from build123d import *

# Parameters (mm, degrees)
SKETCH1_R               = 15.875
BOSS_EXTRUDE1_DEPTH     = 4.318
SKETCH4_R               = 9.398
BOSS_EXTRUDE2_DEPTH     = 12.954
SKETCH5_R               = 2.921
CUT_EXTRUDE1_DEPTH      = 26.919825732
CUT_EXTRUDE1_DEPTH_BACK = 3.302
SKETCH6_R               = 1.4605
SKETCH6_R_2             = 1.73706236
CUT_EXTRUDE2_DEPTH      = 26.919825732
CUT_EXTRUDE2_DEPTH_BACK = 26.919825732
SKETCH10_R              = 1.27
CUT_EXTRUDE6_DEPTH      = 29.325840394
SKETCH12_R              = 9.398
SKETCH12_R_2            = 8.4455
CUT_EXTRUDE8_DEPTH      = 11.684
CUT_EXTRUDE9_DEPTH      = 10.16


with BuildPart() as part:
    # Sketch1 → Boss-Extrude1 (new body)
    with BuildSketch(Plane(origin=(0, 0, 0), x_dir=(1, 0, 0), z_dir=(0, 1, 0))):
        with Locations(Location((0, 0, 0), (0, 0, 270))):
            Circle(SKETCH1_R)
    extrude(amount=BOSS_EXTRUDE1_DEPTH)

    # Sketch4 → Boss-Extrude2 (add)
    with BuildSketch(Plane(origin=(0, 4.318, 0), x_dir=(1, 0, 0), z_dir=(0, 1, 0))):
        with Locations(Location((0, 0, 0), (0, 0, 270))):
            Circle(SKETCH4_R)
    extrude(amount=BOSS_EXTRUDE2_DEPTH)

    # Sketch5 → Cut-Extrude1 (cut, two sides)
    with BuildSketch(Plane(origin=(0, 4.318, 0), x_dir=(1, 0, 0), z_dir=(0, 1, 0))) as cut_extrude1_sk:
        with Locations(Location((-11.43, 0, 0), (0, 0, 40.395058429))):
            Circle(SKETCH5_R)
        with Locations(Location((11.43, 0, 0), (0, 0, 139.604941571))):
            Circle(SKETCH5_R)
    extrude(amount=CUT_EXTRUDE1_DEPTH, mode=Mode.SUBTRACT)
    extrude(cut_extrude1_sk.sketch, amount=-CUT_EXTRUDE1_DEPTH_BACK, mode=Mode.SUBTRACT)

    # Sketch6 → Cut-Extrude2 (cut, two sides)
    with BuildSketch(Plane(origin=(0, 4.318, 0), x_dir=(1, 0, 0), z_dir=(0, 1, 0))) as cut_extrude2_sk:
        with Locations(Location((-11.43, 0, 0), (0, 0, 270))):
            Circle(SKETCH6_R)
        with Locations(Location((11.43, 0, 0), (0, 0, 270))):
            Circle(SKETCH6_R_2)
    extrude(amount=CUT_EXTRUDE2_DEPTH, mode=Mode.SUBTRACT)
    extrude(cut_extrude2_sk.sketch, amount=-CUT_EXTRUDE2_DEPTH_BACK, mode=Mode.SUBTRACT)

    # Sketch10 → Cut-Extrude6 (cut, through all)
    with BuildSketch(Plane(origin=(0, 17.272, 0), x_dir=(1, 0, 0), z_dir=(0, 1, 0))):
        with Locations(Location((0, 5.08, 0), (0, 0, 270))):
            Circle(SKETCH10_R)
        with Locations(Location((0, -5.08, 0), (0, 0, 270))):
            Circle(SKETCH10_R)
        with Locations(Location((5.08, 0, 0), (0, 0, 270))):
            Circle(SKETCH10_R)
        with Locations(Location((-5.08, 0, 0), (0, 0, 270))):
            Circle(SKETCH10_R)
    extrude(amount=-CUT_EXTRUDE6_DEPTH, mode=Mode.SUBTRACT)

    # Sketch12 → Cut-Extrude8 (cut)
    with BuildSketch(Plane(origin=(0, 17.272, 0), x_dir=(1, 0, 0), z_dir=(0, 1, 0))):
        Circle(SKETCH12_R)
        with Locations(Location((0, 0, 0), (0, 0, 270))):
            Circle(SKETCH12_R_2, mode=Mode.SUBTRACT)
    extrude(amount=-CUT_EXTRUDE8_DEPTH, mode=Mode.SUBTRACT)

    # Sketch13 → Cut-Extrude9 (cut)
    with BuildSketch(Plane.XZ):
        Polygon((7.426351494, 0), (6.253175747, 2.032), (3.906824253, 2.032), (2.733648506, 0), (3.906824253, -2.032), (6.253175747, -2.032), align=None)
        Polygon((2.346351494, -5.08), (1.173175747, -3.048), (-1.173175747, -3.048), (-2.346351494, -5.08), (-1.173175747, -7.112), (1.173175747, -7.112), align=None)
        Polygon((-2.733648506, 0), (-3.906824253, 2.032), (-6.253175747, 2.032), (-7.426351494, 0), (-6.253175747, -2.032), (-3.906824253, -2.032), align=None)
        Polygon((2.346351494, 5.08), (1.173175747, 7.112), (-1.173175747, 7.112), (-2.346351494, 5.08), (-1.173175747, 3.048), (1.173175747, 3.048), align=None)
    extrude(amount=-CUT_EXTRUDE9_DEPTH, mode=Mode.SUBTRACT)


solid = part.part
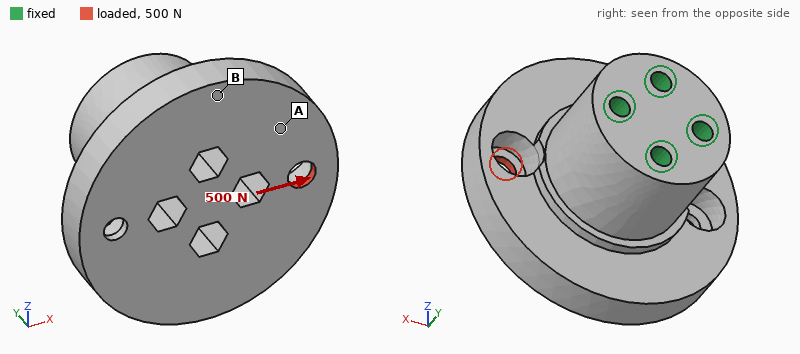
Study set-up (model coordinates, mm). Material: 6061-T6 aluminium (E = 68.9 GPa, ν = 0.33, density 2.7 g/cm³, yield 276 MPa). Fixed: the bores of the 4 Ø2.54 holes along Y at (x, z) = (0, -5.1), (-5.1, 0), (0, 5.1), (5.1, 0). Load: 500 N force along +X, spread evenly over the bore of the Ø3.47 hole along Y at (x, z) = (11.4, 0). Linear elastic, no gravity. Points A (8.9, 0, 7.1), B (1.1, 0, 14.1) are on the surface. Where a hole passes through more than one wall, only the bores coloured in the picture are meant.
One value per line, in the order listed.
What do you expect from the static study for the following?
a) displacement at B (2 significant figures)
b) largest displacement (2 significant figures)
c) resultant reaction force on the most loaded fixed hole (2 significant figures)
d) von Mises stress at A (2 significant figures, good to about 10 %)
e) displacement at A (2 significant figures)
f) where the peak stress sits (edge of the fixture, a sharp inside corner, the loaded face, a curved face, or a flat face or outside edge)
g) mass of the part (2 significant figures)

3.8 µm
14 µm
420 N
13 MPa
5.8 µm
a sharp inside corner
15 g
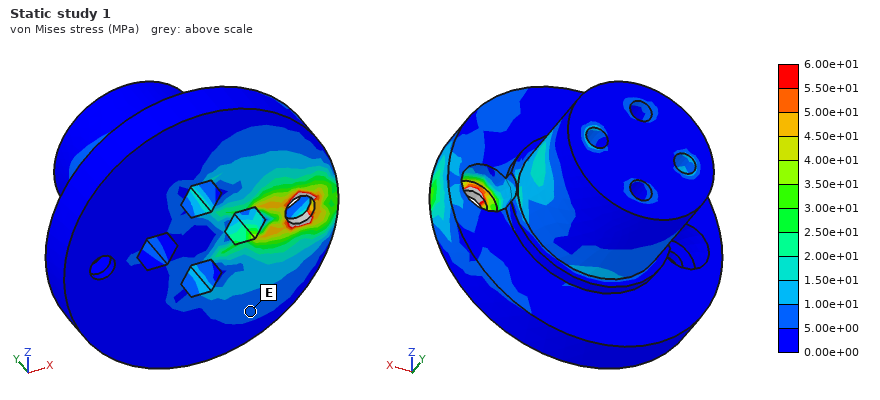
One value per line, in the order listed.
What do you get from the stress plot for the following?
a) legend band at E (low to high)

5.00e+00 to 1.00e+01 MPa
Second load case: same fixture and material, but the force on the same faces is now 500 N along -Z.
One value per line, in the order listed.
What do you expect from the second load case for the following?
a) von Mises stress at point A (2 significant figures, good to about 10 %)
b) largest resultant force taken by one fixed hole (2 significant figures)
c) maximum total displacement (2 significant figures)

11 MPa
470 N
13 µm
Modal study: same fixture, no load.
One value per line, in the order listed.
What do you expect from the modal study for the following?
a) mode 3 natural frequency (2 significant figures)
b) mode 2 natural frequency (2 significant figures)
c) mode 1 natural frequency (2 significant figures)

19 kHz
18 kHz
18 kHz
